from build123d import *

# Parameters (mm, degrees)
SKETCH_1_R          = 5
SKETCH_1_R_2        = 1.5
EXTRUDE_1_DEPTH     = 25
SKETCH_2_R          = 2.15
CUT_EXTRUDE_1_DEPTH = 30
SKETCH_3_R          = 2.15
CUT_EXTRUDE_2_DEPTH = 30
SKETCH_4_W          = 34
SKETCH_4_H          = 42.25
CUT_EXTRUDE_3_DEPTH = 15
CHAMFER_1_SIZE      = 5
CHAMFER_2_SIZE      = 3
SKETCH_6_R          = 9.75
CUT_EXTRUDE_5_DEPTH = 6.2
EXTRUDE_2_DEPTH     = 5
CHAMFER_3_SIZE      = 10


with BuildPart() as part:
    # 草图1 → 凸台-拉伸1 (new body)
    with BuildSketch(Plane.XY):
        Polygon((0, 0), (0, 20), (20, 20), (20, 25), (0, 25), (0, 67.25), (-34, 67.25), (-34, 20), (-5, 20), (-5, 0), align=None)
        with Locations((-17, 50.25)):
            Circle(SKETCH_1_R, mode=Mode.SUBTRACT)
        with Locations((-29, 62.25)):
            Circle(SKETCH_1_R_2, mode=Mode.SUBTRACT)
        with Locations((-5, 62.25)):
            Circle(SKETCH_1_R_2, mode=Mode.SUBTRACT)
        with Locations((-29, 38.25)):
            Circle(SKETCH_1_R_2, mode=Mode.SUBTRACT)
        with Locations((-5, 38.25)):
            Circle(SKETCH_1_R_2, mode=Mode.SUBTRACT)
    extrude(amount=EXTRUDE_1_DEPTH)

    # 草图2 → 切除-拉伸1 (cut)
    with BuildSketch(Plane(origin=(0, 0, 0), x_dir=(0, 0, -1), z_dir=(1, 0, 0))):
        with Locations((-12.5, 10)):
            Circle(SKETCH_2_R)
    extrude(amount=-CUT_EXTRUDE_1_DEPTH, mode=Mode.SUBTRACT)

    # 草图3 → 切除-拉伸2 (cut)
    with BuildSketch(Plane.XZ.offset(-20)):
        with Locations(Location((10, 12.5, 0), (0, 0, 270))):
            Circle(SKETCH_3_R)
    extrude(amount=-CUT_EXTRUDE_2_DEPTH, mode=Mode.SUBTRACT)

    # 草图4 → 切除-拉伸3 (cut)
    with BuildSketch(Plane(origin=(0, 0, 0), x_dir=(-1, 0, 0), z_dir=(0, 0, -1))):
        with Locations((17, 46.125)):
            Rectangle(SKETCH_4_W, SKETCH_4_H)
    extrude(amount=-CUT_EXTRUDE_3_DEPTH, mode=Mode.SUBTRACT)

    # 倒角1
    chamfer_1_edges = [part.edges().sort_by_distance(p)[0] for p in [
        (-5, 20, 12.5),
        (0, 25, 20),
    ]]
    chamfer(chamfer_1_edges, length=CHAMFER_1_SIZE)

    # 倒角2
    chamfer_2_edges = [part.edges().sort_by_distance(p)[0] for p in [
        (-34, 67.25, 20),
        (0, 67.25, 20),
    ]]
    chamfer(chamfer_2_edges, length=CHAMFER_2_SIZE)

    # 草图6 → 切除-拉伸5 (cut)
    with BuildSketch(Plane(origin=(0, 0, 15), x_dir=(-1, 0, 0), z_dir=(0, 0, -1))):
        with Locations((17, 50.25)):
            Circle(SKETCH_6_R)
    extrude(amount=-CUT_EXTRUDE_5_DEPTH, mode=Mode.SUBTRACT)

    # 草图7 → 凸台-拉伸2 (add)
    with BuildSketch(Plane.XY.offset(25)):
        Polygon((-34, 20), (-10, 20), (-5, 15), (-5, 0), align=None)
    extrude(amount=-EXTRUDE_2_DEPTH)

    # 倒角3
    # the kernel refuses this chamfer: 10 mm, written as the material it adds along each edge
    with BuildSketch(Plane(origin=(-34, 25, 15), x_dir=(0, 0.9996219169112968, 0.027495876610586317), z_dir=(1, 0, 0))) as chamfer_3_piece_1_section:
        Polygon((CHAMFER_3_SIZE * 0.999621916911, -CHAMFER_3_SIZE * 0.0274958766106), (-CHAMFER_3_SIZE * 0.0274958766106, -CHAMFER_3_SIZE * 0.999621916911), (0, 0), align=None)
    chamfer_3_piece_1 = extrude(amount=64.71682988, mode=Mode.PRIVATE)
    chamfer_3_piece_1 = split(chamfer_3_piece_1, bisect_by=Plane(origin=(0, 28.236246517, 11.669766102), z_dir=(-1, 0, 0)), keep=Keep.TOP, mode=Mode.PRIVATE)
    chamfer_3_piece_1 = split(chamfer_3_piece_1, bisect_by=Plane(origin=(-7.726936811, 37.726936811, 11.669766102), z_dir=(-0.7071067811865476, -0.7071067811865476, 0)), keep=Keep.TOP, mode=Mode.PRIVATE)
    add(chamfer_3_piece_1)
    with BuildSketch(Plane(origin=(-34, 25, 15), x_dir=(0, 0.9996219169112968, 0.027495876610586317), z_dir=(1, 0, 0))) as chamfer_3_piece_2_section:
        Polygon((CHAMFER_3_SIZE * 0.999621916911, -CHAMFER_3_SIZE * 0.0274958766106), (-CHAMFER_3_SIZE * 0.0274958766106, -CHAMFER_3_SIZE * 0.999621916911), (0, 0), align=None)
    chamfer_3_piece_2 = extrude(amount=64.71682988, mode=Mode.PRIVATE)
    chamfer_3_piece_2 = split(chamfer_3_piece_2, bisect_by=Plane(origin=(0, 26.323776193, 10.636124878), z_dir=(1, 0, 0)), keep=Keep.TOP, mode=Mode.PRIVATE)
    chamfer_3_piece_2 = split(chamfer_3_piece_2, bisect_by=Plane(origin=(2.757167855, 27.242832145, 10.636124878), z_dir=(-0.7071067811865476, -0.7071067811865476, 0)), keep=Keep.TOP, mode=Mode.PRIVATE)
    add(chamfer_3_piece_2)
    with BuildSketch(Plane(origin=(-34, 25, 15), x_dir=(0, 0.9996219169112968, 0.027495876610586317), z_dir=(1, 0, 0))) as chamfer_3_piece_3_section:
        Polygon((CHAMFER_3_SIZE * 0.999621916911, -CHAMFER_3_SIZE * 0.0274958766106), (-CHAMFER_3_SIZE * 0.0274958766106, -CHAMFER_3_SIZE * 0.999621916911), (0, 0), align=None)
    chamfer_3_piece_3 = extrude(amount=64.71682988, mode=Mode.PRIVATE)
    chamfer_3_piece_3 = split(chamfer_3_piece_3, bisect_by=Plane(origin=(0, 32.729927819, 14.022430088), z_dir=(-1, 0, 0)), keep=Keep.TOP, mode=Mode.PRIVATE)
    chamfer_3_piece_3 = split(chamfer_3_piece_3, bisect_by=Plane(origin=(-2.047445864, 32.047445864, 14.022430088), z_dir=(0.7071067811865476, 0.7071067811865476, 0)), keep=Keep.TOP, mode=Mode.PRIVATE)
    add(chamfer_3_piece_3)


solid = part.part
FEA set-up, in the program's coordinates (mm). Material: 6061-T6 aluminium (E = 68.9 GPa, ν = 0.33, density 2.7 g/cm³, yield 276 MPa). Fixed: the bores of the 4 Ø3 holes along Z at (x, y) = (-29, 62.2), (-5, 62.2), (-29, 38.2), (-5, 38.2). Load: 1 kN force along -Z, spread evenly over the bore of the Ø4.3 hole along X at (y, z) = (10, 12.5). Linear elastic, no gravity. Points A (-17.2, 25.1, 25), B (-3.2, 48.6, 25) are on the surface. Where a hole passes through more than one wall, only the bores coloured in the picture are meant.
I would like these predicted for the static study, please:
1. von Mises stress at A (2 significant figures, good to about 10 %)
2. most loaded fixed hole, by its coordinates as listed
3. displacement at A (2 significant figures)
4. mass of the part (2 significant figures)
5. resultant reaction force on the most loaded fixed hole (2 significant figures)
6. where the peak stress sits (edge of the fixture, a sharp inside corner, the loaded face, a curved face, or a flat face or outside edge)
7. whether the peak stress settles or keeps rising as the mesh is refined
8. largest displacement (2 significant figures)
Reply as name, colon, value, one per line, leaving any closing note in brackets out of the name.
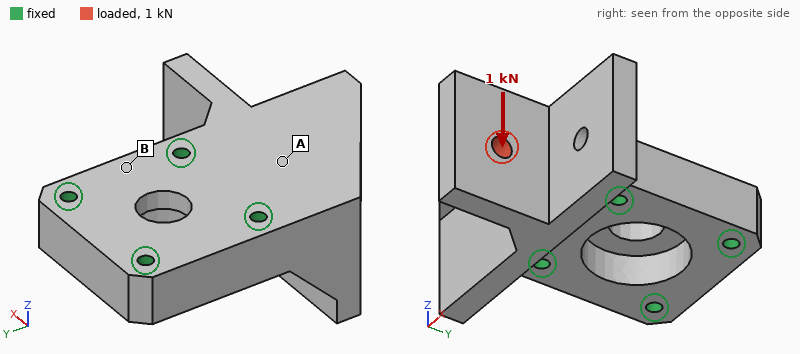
von Mises stress at A: 20 MPa
most loaded fixed hole, by its coordinates as listed: (-5, 38.2)
displacement at A: 17 µm
mass of the part: 66 g
resultant reaction force on the most loaded fixed hole: 1.1 kN
where the peak stress sits: edge of the fixture
whether the peak stress settles or keeps rising as the mesh is refined: keeps rising
largest displacement: 84 µm
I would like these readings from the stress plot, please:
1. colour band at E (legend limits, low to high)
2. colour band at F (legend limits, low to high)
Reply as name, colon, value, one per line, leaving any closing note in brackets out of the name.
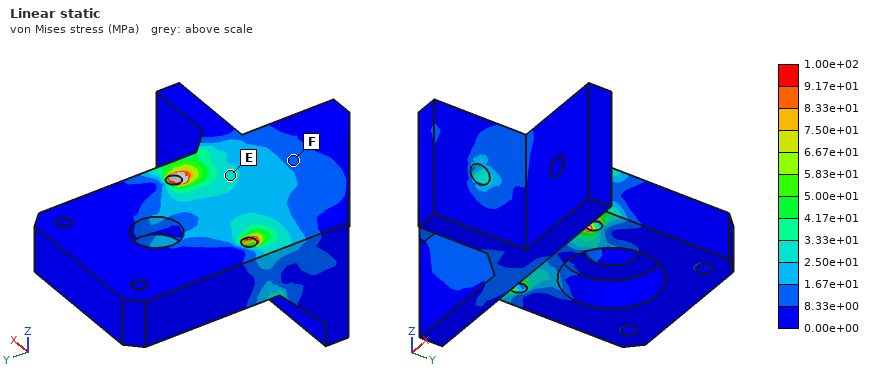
colour band at E: 2.50e+01 to 3.33e+01 MPa
colour band at F: 8.33e+00 to 1.67e+01 MPa
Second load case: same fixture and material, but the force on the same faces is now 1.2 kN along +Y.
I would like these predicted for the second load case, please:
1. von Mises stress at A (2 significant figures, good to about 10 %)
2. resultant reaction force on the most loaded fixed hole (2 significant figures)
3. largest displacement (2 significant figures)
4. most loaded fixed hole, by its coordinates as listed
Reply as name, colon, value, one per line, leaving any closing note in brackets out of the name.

von Mises stress at A: 6.6 MPa
resultant reaction force on the most loaded fixed hole: 1.2 kN
largest displacement: 29 µm
most loaded fixed hole, by its coordinates as listed: (-5, 38.2)
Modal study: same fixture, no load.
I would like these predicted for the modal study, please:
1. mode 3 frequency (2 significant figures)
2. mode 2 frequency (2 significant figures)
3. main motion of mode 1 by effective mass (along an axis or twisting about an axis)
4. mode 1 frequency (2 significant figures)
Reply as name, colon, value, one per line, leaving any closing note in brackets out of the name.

mode 3 frequency: 11 kHz
mode 2 frequency: 9200 Hz
main motion of mode 1 by effective mass: along Z
mode 1 frequency: 5200 Hz
